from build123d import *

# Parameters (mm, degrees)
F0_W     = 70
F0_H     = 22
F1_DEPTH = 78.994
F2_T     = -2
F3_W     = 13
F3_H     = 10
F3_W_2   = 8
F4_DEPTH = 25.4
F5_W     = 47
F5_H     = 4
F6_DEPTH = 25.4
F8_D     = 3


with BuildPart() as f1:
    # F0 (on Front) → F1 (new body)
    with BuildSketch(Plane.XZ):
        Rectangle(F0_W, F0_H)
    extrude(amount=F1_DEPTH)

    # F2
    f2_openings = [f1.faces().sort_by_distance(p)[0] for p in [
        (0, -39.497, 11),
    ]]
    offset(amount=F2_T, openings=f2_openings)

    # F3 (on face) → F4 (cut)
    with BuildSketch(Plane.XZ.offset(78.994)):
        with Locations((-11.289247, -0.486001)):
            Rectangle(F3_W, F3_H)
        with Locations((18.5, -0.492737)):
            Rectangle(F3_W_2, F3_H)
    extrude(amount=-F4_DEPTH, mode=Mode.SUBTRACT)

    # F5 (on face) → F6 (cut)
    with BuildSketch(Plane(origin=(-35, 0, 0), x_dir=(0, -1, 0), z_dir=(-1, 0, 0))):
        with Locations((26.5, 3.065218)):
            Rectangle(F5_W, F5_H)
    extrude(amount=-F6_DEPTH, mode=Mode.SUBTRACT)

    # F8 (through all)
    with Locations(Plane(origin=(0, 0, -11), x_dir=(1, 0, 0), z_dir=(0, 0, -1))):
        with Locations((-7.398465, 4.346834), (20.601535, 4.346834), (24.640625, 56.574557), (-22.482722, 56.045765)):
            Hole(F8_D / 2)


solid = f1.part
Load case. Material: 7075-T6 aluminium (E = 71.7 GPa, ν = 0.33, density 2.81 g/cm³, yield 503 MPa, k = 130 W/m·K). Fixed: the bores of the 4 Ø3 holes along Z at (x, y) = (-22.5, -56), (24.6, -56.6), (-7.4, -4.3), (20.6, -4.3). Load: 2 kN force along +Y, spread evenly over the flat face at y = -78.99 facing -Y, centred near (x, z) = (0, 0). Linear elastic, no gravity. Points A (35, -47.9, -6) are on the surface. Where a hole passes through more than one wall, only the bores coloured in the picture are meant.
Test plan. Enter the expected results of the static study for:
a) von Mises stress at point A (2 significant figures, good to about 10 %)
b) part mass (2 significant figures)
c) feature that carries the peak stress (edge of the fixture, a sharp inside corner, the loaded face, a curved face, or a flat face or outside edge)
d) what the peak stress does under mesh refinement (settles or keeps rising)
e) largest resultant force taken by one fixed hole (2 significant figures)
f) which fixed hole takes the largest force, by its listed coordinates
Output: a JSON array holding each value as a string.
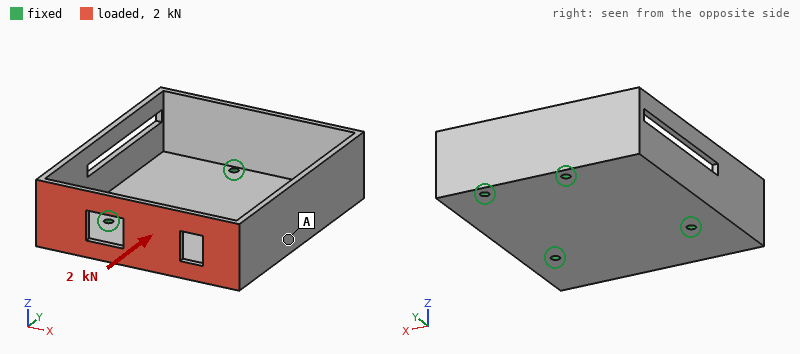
["33 MPa", "61 g", "edge of the fixture", "keeps rising", "830 N", "(-22.5, -56)"]
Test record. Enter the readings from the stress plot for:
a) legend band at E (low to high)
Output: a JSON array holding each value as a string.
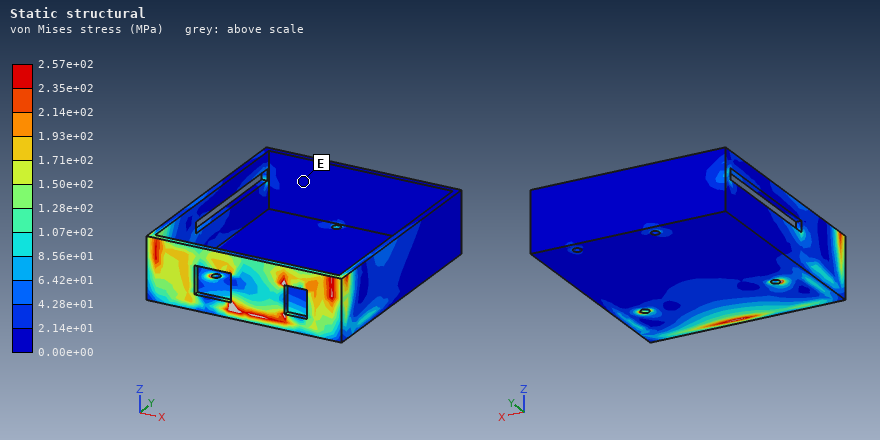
["0.00e+00 to 2.14e+01 MPa"]
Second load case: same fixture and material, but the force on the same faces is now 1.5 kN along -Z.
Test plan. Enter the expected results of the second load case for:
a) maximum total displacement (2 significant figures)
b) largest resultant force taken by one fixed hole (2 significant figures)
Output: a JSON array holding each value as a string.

["0.48 mm", "1.1 kN"]
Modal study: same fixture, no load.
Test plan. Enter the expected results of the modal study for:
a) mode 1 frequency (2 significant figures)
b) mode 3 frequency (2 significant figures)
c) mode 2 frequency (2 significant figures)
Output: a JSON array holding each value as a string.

["2400 Hz", "2900 Hz", "2800 Hz"]
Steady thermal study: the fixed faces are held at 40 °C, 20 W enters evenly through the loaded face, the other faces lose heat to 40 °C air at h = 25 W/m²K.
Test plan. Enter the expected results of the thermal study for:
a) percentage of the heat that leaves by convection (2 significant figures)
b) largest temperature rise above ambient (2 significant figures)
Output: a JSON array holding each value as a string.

["20 %", "33 K"]
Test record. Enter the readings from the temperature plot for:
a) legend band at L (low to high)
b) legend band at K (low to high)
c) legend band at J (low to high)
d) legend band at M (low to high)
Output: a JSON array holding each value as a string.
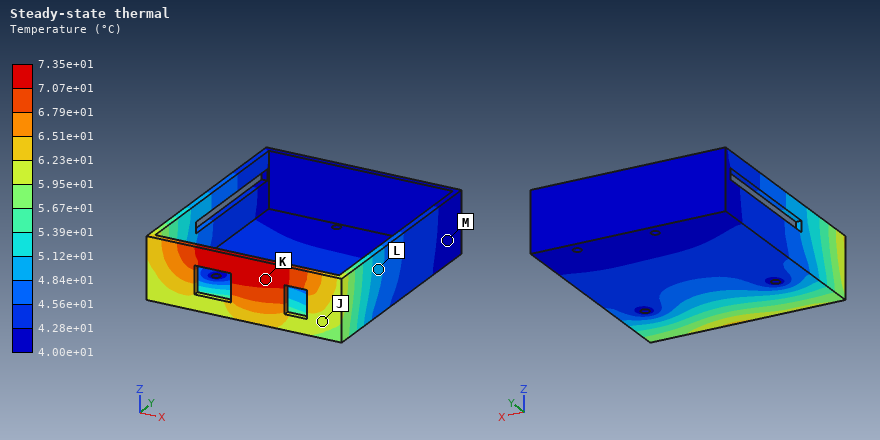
["4.84e+01 to 5.12e+01 °C", "7.07e+01 to 7.35e+01 °C", "5.95e+01 to 6.23e+01 °C", "4.00e+01 to 4.28e+01 °C"]
